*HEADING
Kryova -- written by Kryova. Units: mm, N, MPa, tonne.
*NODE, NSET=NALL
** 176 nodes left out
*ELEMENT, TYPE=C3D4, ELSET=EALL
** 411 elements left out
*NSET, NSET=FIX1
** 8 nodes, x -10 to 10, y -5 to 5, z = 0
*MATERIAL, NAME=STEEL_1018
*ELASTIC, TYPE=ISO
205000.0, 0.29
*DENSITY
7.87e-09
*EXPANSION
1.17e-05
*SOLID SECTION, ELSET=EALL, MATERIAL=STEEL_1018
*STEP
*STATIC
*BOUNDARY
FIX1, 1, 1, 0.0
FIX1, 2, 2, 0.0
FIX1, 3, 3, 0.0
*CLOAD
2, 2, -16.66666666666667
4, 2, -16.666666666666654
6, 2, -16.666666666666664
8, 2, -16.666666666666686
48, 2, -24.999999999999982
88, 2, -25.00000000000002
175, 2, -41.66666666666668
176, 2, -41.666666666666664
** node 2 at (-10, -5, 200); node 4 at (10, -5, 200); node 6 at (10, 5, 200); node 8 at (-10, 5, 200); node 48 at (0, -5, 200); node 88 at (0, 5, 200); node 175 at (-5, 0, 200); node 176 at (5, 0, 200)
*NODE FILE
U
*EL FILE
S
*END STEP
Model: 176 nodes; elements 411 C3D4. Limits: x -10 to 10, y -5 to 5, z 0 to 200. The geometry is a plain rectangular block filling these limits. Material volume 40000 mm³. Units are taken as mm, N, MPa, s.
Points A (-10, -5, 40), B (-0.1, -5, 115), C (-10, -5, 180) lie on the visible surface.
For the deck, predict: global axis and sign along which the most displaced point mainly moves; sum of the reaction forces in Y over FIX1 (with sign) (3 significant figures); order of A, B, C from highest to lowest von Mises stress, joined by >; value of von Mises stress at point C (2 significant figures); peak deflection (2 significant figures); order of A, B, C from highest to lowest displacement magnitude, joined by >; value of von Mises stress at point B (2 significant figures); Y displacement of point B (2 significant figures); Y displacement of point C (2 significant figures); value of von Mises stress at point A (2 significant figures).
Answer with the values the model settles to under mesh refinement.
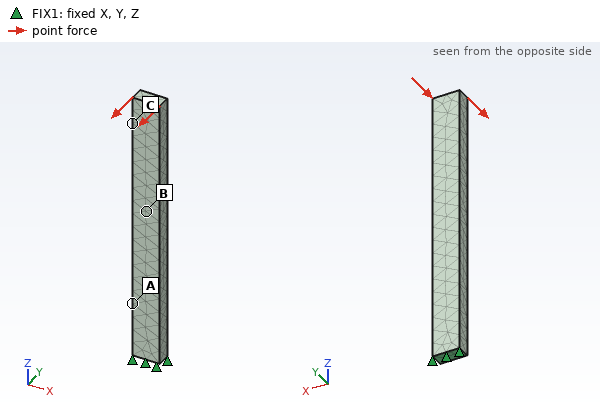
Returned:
-Y
200 N
A > B > C
12 MPa
1.6 mm
C > B > A
51 MPa
-0.62 mm
-1.3 mm
96 MPa
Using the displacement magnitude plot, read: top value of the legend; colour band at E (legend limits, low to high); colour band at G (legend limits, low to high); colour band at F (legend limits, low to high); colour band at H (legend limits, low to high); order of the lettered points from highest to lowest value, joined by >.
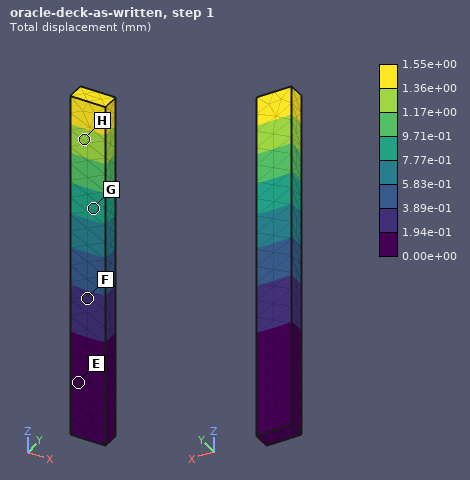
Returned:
1.55e+00 mm
0.00e+00 to 1.94e-01 mm
7.77e-01 to 9.71e-01 mm
1.94e-01 to 3.89e-01 mm
1.17e+00 to 1.36e+00 mm
H > G > F > E
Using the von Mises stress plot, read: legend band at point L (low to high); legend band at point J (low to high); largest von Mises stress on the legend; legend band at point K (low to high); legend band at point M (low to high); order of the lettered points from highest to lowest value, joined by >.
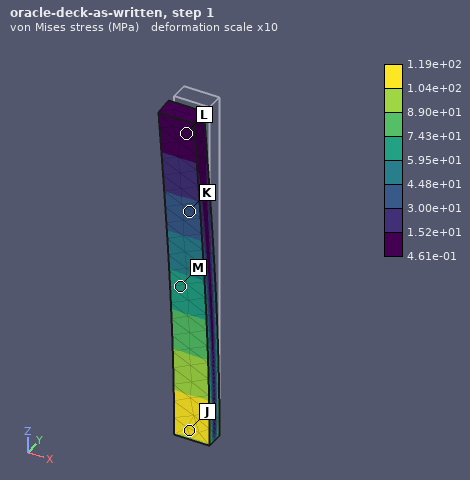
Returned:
4.61e-01 to 1.52e+01 MPa
1.04e+02 to 1.19e+02 MPa
1.19e+02 MPa
3.00e+01 to 4.48e+01 MPa
5.95e+01 to 7.43e+01 MPa
J > M > K > L
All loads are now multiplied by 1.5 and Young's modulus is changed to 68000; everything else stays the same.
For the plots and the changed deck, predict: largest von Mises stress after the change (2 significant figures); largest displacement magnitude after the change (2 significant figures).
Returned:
180 MPa
7.0 mm
